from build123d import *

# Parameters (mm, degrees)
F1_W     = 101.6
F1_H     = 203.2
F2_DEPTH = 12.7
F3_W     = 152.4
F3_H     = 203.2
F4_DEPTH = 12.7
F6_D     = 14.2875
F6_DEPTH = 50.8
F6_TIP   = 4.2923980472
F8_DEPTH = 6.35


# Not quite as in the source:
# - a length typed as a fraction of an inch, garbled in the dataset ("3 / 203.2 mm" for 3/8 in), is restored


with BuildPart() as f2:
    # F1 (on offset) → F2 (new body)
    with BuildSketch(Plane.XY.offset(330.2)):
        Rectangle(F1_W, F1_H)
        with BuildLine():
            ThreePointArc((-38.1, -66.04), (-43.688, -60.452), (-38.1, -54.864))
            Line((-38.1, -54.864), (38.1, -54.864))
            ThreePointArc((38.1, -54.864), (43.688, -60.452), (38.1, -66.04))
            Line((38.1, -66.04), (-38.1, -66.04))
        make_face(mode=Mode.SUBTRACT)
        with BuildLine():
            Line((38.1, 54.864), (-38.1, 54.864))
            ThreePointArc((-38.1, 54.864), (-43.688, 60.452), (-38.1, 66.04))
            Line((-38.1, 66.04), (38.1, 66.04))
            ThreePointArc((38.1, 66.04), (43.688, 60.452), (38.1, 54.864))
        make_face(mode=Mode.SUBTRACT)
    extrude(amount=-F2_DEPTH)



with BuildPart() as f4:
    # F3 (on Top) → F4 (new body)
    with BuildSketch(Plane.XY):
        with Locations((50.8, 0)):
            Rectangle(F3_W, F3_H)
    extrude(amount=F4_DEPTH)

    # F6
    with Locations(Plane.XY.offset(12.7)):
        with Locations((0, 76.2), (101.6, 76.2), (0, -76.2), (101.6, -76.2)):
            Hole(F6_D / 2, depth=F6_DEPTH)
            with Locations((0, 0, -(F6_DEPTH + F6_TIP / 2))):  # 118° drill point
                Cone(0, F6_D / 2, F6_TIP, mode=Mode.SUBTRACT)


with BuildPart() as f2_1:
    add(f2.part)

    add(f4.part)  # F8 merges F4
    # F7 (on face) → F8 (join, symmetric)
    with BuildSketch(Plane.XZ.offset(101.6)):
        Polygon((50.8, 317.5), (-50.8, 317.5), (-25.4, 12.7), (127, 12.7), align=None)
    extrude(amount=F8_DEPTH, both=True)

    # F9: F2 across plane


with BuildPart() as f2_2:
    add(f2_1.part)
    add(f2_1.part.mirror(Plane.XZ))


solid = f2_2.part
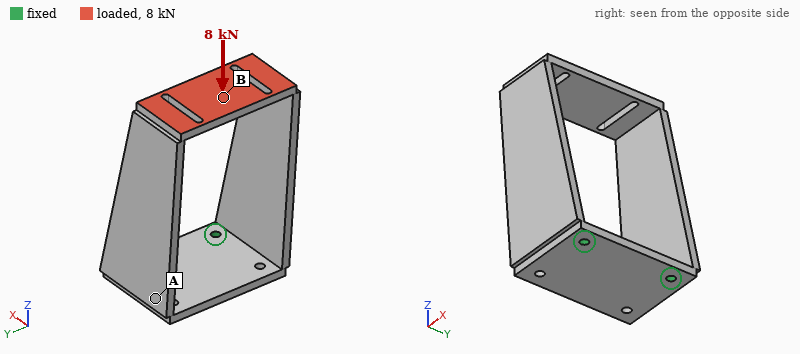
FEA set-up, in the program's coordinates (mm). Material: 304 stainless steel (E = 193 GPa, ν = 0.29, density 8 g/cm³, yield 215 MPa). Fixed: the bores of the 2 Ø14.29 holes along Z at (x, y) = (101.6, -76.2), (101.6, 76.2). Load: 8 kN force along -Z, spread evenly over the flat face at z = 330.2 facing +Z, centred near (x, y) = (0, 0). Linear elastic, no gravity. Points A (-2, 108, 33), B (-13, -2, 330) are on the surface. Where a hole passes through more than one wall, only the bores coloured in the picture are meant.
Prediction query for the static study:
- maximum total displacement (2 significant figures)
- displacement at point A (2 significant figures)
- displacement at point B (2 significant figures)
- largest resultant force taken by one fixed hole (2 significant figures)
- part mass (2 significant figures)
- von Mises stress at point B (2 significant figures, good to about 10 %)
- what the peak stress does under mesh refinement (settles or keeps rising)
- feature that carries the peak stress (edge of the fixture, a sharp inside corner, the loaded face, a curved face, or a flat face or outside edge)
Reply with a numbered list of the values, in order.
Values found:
1. 0.94 mm
2. 0.26 mm
3. 0.88 mm
4. 4.0 kN
5. 13 kg
6. 35 MPa
7. keeps rising
8. edge of the fixture
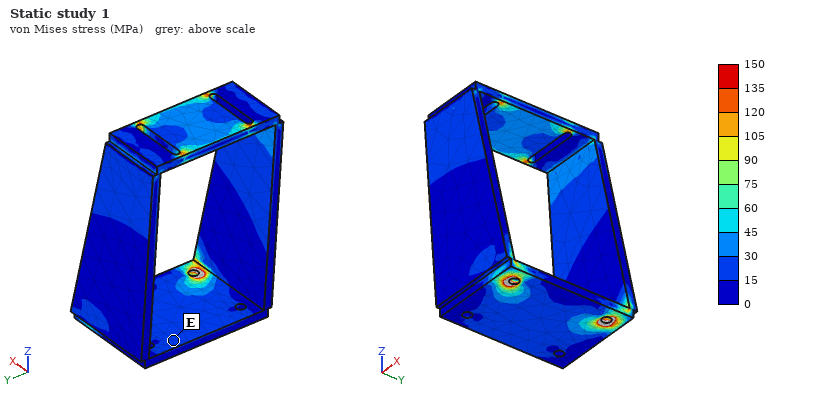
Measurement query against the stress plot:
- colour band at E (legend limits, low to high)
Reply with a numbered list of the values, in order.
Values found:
1. 15 to 30 MPa
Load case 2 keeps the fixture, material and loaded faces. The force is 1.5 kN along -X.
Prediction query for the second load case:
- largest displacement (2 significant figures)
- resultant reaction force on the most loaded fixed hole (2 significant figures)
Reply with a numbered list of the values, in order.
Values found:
1. 0.51 mm
2. 760 N
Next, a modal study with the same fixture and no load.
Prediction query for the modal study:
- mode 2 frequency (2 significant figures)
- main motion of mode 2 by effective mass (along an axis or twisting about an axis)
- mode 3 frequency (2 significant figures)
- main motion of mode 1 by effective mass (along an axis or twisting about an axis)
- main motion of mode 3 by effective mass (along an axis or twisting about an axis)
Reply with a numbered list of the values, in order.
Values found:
1. 130 Hz
2. along X
3. 250 Hz
4. along Y
5. twisting about Z
